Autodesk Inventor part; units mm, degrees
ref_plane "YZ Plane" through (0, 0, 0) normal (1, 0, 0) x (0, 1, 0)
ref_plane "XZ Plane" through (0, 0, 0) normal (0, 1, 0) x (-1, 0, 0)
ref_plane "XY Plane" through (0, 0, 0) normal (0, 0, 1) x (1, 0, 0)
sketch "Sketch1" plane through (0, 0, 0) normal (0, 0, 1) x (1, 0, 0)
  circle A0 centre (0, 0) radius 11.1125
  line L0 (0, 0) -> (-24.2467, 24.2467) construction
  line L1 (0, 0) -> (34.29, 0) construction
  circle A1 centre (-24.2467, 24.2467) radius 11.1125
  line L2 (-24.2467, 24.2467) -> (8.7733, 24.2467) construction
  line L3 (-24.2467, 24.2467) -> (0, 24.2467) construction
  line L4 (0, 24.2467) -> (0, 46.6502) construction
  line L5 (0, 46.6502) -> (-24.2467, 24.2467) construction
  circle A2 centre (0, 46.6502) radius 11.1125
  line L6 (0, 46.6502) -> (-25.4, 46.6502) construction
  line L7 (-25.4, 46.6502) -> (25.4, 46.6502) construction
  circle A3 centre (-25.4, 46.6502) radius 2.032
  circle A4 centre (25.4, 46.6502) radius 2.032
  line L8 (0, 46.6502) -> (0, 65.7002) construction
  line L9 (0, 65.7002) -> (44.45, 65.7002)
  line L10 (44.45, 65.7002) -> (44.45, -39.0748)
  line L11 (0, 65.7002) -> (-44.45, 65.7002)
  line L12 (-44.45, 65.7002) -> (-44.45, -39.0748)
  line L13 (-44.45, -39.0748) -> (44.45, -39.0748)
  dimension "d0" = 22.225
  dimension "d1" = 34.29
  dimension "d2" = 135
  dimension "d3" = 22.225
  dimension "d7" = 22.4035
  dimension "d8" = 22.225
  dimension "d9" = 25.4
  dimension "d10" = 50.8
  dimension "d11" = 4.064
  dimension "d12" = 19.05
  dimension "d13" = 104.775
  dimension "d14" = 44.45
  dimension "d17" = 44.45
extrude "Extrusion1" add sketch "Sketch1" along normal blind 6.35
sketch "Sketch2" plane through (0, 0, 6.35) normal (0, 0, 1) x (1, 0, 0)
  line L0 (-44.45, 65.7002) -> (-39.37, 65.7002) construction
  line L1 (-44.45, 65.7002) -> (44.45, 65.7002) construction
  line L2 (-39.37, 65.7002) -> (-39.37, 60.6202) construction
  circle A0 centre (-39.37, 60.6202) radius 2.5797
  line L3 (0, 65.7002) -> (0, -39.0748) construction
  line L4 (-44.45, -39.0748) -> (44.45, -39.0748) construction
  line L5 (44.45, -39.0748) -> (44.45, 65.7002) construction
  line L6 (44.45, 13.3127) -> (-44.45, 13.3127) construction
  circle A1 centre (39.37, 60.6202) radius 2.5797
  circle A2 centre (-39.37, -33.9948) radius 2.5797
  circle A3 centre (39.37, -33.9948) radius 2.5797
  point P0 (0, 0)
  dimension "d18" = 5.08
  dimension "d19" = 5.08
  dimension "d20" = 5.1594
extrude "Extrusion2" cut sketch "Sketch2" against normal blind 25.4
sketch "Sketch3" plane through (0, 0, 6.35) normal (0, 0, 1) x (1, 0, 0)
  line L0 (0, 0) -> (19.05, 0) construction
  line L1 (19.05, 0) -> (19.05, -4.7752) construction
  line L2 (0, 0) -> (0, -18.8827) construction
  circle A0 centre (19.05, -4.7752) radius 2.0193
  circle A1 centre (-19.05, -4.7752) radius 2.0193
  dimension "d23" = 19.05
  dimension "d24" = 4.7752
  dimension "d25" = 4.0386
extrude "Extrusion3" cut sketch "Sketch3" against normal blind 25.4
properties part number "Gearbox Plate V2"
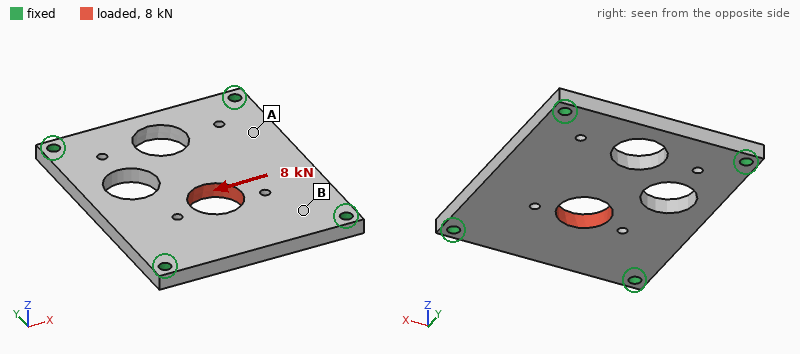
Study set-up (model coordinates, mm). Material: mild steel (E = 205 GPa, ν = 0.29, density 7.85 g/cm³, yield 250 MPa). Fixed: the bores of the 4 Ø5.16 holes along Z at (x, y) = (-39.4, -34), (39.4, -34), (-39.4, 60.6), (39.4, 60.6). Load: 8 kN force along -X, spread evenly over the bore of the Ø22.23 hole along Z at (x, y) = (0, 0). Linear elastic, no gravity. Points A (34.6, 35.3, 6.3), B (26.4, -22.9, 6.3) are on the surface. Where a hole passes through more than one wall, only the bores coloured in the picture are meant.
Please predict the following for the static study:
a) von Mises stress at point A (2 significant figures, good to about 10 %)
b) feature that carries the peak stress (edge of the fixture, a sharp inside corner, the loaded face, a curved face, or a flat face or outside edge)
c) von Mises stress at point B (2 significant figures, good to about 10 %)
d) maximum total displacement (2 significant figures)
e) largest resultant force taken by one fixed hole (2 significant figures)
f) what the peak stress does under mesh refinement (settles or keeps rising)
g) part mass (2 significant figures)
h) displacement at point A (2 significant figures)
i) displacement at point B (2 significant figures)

8.3 MPa
edge of the fixture
22 MPa
8.2 µm
3.2 kN
keeps rising
400 g
4.0 µm
2.9 µm
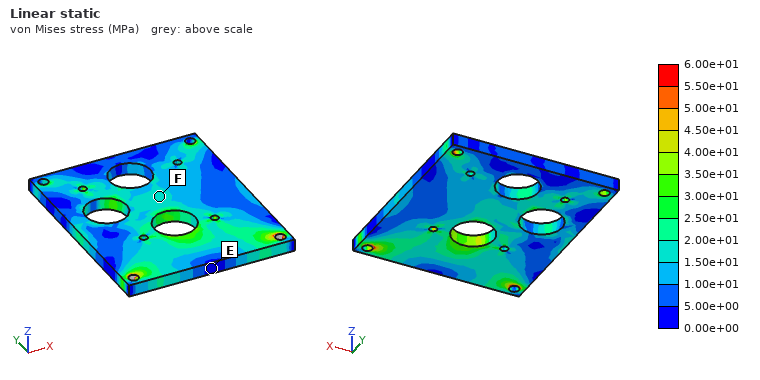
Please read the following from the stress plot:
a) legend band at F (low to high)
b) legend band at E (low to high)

1.50e+01 to 2.00e+01 MPa
0.00e+00 to 5.00e+00 MPa
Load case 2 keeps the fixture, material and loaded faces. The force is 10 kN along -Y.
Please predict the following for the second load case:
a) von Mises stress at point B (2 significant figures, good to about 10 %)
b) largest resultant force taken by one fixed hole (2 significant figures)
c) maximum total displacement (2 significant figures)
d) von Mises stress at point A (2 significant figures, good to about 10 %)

24 MPa
3.4 kN
8.8 µm
13 MPa
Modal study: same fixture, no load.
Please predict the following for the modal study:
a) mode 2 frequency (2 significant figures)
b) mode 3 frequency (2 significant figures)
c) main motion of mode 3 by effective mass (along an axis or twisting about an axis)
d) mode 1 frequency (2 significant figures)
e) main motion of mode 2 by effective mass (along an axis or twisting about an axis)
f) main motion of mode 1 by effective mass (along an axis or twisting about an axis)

4200 Hz
5200 Hz
twisting about X
2600 Hz
twisting about Y
along Z
